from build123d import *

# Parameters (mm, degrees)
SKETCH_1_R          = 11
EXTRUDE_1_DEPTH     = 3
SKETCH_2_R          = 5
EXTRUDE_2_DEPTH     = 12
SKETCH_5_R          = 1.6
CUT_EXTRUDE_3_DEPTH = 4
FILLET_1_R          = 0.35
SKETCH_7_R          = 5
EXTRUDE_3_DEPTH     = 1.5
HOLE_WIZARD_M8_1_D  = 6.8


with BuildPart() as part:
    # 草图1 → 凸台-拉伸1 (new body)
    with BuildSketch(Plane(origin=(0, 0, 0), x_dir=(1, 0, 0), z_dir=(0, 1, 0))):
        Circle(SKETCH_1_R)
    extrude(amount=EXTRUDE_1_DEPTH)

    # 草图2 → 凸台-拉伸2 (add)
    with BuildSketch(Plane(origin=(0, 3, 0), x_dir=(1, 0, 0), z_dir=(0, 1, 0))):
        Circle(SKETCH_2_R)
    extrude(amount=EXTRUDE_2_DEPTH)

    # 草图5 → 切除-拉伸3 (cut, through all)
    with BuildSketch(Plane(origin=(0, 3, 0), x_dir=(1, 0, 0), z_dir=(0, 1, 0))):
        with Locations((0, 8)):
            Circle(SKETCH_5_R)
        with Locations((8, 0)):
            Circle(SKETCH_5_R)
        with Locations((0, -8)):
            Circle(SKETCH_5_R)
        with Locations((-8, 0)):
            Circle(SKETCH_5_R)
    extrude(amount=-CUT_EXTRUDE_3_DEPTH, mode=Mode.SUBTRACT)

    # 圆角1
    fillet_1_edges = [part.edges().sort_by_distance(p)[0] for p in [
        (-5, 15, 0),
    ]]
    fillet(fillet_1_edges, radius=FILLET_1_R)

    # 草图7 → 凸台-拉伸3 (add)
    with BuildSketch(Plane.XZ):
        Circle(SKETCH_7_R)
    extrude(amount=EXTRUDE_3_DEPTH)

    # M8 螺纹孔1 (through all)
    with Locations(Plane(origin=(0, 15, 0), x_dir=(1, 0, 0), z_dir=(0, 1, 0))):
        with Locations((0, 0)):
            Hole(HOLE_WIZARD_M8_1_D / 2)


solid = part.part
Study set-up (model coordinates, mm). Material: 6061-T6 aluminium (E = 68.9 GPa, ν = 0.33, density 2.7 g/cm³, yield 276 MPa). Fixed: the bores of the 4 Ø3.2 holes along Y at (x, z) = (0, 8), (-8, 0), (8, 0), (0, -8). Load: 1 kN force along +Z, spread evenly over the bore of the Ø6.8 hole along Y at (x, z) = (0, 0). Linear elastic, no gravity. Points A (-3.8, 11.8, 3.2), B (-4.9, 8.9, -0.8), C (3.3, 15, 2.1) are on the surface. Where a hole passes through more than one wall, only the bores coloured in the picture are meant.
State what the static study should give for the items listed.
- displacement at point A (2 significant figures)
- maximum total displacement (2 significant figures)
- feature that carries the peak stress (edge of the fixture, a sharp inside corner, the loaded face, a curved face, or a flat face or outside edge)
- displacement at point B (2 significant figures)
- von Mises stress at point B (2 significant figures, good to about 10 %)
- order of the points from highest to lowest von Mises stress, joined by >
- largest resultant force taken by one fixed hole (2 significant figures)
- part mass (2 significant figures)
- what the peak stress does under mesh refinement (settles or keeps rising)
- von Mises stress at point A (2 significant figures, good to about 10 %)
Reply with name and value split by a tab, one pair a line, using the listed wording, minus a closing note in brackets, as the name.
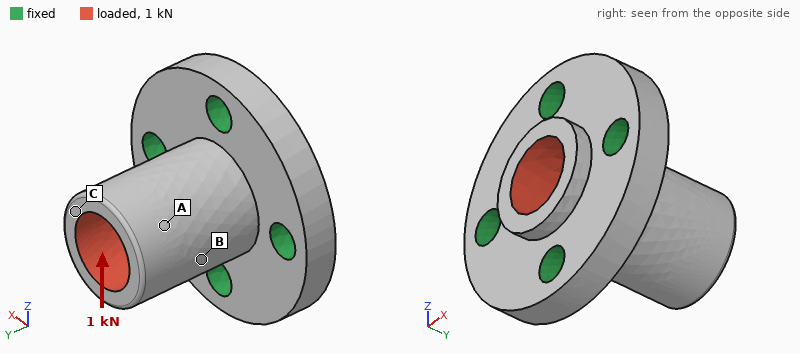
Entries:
displacement at point A	17 µm
maximum total displacement	22 µm
feature that carries the peak stress	edge of the fixture
displacement at point B	11 µm
von Mises stress at point B	26 MPa
order of the points from highest to lowest von Mises stress, joined by >	B > A > C
largest resultant force taken by one fixed hole	490 N
part mass	4.1 g
what the peak stress does under mesh refinement	keeps rising
von Mises stress at point A	12 MPa
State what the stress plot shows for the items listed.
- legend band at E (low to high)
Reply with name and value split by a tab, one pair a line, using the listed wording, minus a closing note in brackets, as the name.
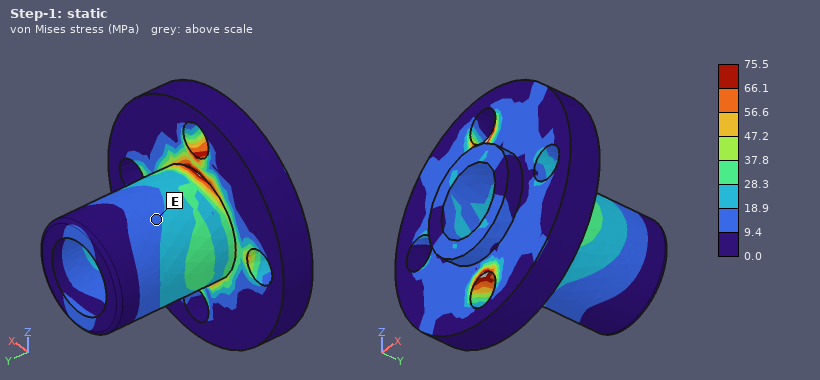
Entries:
legend band at E	9.4 to 18.9 MPa
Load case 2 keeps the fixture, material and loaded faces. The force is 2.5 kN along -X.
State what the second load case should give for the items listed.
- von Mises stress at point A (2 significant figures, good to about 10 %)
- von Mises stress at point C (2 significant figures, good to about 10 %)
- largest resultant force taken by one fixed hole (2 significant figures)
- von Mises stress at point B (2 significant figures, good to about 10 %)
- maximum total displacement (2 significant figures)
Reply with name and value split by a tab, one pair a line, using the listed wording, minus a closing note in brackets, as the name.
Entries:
von Mises stress at point A	27 MPa
von Mises stress at point C	23 MPa
largest resultant force taken by one fixed hole	1.2 kN
von Mises stress at point B	35 MPa
maximum total displacement	55 µm
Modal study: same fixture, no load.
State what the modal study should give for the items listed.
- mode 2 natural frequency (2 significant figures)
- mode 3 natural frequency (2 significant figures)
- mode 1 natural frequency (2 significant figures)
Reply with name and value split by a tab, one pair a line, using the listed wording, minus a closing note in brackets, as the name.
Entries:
mode 2 natural frequency	29 kHz
mode 3 natural frequency	59 kHz
mode 1 natural frequency	29 kHz
